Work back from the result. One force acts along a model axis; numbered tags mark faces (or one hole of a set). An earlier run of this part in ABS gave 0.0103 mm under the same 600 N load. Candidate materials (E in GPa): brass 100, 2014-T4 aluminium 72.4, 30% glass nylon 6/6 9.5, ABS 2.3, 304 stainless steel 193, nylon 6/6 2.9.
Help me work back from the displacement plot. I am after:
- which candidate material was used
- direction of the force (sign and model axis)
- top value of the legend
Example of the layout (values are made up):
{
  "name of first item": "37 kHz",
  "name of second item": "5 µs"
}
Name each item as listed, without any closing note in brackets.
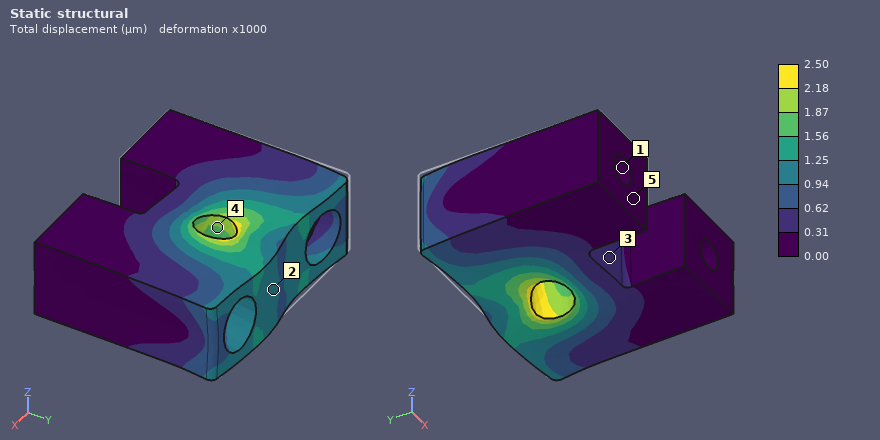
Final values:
{
  "which candidate material was used": "30% glass nylon 6/6",
  "direction of the force": "+X",
  "top value of the legend": "2.50 µm"
}
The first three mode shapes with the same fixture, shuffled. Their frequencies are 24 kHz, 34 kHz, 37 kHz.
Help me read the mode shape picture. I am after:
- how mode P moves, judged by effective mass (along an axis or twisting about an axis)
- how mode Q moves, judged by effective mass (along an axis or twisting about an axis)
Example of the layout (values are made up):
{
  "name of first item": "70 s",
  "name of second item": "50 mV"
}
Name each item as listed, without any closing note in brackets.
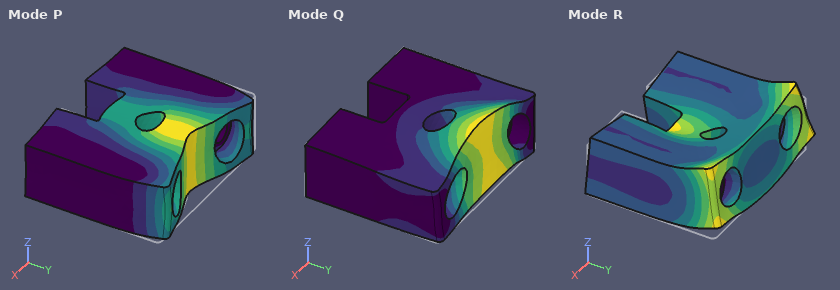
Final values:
{
  "how mode P moves, judged by effective mass": "along Y",
  "how mode Q moves, judged by effective mass": "along Z"
}
